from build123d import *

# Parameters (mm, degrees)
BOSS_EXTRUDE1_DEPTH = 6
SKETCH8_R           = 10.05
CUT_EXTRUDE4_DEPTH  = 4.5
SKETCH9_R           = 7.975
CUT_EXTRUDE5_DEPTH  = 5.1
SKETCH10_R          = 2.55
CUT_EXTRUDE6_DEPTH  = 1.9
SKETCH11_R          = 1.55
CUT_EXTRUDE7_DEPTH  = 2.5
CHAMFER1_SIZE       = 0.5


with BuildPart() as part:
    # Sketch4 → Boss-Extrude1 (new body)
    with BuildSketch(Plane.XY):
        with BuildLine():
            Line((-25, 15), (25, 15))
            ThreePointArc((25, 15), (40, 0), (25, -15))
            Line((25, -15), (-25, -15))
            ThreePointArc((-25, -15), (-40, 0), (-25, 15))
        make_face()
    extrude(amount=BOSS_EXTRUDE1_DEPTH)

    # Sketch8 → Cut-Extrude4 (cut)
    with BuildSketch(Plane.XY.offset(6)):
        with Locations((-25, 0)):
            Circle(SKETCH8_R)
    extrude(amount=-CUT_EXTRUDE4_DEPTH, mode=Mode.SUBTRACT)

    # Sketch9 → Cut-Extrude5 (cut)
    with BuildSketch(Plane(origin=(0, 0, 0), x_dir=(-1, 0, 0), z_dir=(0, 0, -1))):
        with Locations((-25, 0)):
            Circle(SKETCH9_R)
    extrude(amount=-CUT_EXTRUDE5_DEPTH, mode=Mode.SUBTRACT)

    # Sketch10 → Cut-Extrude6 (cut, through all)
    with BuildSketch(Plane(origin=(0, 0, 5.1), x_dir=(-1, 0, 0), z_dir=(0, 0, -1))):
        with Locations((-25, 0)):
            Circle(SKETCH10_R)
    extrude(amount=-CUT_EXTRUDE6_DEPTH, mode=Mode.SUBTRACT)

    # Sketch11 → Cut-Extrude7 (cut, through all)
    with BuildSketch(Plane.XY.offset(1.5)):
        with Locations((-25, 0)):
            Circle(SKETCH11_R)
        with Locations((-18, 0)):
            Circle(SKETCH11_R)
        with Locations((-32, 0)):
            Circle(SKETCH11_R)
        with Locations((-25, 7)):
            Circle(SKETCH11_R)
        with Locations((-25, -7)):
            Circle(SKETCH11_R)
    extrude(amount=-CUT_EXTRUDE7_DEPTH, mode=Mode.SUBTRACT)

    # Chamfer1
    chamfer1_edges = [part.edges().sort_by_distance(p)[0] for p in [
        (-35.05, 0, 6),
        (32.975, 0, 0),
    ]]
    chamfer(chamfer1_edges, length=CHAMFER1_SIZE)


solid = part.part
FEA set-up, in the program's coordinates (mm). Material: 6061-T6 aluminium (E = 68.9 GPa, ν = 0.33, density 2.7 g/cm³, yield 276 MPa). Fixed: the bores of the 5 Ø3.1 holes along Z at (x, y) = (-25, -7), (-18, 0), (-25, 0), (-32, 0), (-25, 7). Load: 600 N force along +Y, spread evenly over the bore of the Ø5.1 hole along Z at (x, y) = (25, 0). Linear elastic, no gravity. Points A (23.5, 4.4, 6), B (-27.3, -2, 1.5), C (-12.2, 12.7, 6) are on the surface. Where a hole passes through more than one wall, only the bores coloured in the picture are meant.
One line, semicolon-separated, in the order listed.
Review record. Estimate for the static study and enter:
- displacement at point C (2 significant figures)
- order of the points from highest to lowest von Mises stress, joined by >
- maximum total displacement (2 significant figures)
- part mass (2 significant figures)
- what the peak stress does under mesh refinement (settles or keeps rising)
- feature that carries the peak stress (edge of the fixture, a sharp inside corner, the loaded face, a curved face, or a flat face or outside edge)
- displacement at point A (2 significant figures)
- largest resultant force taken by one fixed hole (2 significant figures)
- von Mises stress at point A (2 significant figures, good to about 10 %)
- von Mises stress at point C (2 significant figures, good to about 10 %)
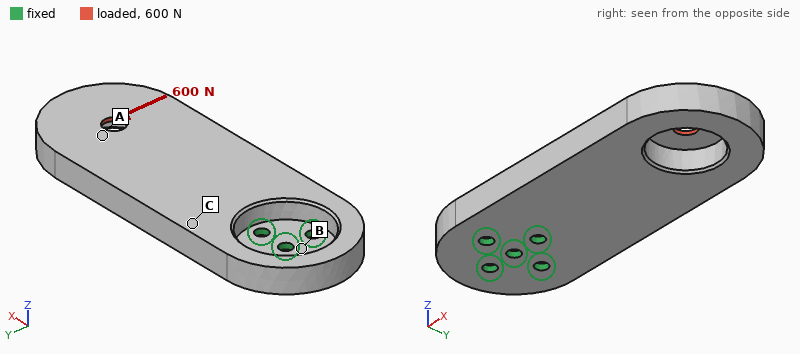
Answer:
21 µm; A > C > B; 96 µm; 29 g; keeps rising; edge of the fixture; 72 µm; 1.1 kN; 39 MPa; 21 MPa
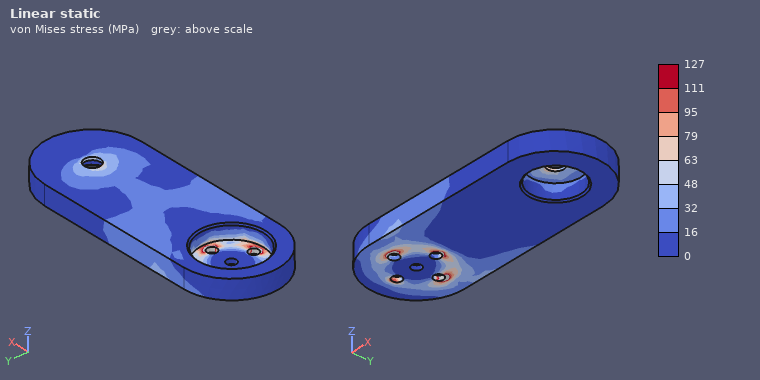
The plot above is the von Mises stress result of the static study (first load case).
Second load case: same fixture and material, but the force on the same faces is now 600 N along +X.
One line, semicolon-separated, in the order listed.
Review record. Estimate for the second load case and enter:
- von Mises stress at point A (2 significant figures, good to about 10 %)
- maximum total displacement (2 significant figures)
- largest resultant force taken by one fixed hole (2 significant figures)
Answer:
26 MPa; 0.15 mm; 260 N
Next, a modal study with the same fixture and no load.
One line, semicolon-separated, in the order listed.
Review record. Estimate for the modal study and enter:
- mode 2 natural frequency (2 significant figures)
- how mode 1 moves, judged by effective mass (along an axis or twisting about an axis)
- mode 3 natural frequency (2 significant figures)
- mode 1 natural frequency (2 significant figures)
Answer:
4100 Hz; along Z; 4200 Hz; 1100 Hz
